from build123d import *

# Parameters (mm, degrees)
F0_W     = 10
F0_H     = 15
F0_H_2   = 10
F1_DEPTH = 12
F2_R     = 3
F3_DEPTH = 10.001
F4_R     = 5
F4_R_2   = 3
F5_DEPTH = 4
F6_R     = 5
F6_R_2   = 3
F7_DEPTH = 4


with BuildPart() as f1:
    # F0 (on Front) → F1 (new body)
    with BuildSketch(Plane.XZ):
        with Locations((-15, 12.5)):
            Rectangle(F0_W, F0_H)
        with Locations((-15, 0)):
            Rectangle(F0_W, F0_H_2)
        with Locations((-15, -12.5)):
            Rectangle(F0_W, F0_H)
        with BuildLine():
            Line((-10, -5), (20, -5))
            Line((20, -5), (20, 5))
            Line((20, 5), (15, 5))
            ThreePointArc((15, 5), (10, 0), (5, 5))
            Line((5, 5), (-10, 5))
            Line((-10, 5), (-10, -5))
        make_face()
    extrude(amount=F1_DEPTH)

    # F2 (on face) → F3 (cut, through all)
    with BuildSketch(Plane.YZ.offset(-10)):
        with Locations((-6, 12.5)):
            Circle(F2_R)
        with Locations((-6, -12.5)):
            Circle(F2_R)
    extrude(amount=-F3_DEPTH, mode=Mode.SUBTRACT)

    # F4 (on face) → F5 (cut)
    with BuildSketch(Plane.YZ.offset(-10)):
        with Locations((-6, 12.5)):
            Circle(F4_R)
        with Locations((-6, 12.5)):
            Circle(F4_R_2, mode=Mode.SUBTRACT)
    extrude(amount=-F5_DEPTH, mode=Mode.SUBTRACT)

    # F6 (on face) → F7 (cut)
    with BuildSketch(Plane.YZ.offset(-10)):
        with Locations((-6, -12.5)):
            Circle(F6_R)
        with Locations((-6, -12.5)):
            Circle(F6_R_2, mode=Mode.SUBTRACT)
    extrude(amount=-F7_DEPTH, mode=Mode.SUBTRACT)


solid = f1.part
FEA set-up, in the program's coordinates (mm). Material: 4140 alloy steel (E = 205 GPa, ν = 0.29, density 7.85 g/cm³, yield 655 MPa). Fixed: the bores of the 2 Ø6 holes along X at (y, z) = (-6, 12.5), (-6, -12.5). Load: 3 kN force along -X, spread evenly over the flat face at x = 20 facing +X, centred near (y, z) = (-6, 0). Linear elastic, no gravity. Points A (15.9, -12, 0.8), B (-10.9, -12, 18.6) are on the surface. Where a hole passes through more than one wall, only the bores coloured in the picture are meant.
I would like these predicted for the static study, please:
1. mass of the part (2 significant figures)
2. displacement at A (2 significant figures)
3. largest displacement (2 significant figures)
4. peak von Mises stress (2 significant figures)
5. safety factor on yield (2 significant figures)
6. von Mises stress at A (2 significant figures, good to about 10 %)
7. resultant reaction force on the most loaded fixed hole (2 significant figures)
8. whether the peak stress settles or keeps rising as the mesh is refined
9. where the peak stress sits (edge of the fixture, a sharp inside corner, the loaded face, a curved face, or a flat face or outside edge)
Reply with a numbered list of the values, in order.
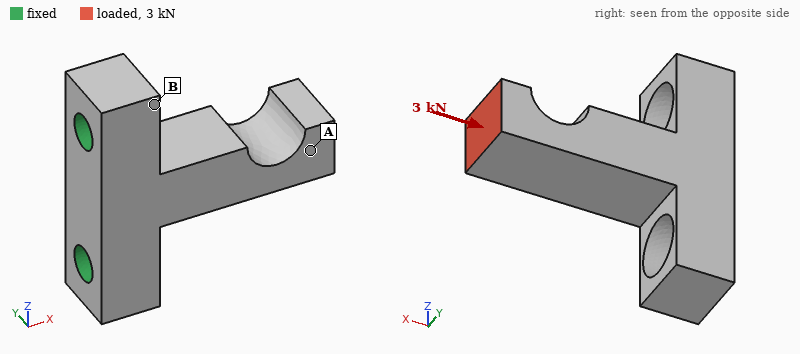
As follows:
1. 55 g
2. 19 µm
3. 33 µm
4. 230 MPa
5. 2.8
6. 57 MPa
7. 1.6 kN
8. settles
9. a curved face
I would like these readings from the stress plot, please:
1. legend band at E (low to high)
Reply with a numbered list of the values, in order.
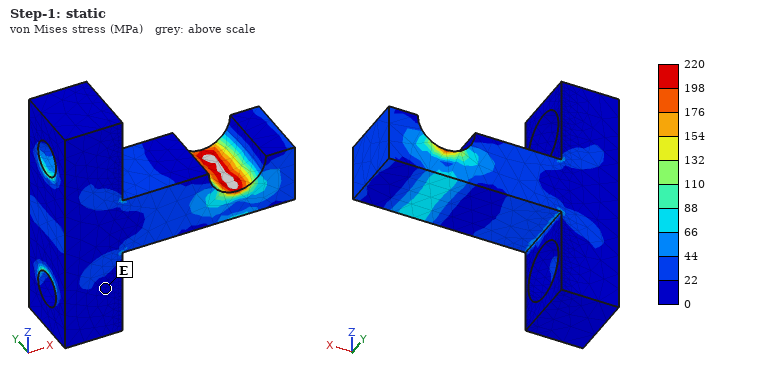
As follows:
1. 0 to 22 MPa
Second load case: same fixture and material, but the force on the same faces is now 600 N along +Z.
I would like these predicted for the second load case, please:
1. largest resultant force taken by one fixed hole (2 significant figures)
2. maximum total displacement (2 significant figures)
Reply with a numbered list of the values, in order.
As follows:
1. 1.2 kN
2. 63 µm
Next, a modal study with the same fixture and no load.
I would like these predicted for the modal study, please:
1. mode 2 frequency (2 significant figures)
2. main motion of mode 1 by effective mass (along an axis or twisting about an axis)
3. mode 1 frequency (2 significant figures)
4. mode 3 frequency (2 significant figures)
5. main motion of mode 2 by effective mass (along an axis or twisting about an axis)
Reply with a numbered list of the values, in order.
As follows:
1. 6800 Hz
2. along Y
3. 5500 Hz
4. 20 kHz
5. along Z
